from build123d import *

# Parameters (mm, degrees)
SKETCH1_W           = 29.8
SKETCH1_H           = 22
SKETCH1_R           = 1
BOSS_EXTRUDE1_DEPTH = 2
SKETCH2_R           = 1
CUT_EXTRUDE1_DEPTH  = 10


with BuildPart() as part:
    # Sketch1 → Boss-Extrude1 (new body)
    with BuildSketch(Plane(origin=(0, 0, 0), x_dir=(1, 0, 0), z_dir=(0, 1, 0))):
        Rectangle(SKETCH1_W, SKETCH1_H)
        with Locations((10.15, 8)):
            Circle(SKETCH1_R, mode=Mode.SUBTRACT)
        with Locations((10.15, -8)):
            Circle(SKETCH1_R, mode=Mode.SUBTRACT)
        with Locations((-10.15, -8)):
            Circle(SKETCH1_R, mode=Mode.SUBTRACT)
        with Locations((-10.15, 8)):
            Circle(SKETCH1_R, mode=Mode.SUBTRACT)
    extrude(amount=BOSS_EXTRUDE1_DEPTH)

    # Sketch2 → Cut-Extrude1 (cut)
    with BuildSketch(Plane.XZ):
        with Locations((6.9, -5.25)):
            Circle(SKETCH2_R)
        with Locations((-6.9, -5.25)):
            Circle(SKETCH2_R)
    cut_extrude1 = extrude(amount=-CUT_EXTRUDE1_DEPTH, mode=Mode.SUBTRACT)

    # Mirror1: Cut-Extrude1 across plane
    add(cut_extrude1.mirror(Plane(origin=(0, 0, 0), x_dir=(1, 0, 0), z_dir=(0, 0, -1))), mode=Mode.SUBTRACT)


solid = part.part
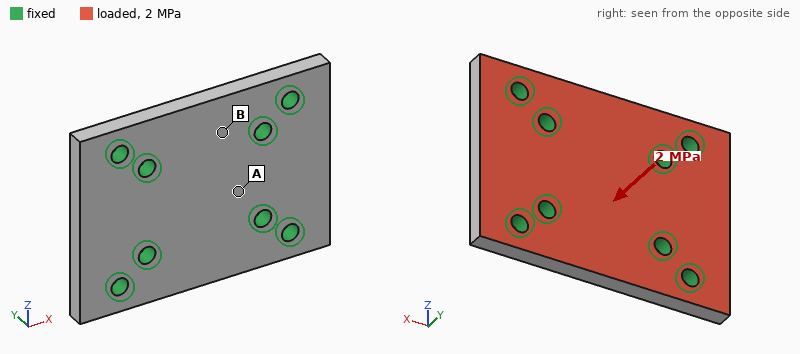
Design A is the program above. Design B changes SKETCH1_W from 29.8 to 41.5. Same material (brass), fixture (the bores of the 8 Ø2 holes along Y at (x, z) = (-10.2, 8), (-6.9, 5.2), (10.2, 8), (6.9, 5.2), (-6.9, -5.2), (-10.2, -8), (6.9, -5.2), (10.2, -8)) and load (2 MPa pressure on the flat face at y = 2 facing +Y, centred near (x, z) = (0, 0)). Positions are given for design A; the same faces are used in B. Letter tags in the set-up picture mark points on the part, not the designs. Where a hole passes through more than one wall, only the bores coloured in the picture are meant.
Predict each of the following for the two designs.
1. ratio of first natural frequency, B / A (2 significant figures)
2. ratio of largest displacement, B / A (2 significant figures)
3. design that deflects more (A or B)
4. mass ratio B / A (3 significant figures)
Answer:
0.33
9.3
B
1.41
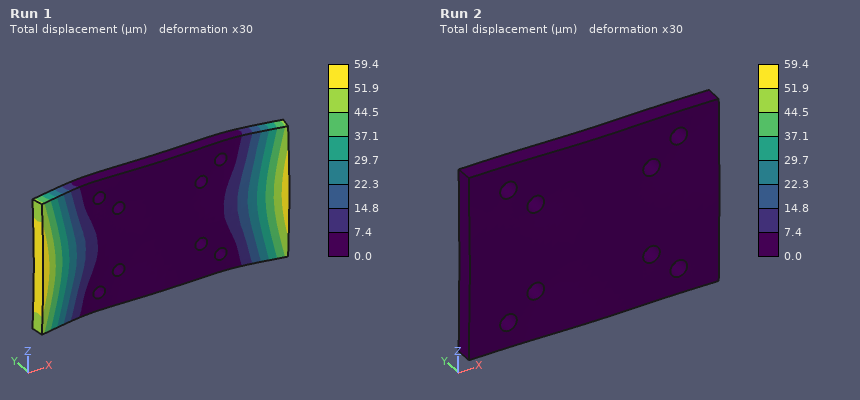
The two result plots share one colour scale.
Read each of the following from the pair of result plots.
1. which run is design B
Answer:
Run 1
